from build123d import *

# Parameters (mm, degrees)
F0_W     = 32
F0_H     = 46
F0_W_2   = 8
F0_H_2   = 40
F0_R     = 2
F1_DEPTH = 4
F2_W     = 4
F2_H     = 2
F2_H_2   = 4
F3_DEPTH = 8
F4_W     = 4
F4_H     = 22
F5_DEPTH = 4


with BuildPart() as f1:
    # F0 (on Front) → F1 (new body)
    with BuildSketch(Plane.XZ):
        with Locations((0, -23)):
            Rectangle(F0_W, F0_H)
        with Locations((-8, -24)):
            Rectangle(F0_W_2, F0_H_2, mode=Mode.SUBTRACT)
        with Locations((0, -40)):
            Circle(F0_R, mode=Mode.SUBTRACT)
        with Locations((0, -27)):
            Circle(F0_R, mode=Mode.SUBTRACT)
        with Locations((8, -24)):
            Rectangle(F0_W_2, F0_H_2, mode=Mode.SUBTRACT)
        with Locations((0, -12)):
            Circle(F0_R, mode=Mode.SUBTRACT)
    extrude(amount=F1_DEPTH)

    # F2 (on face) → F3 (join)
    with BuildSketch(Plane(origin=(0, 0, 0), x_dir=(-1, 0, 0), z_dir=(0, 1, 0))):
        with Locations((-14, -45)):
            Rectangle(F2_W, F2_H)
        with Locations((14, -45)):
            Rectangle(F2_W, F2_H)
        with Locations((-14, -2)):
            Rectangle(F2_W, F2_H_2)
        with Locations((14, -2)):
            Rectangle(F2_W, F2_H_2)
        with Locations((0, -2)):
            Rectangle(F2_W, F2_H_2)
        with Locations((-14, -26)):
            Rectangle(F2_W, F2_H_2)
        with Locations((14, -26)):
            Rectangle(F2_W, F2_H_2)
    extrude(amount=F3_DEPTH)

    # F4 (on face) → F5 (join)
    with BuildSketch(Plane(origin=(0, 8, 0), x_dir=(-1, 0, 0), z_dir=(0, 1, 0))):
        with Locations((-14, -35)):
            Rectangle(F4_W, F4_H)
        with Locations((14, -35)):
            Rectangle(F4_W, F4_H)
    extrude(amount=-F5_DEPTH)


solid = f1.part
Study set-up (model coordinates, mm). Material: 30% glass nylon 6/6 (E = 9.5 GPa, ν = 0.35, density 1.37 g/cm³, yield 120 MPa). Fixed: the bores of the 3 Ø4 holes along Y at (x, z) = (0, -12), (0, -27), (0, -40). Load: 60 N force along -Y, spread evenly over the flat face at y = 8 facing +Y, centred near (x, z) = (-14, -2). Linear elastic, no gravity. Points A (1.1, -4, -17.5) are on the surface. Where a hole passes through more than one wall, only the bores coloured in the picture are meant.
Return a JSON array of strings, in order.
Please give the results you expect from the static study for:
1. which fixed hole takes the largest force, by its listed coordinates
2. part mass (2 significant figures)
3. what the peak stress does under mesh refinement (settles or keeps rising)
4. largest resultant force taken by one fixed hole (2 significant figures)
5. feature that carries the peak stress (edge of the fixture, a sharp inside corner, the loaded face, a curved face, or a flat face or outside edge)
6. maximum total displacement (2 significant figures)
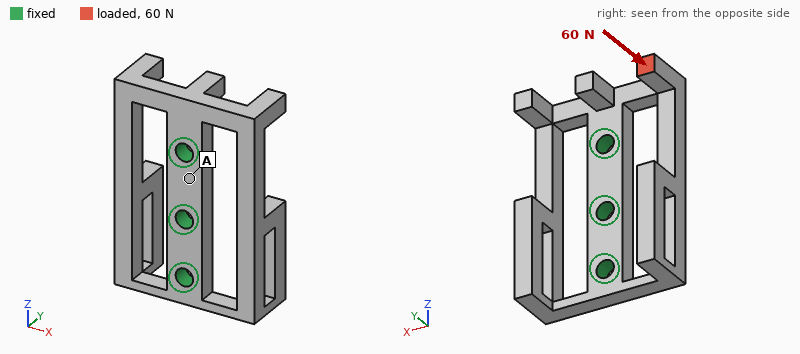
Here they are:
["(0, -12)", "6.1 g", "keeps rising", "61 N", "edge of the fixture", "0.53 mm"]
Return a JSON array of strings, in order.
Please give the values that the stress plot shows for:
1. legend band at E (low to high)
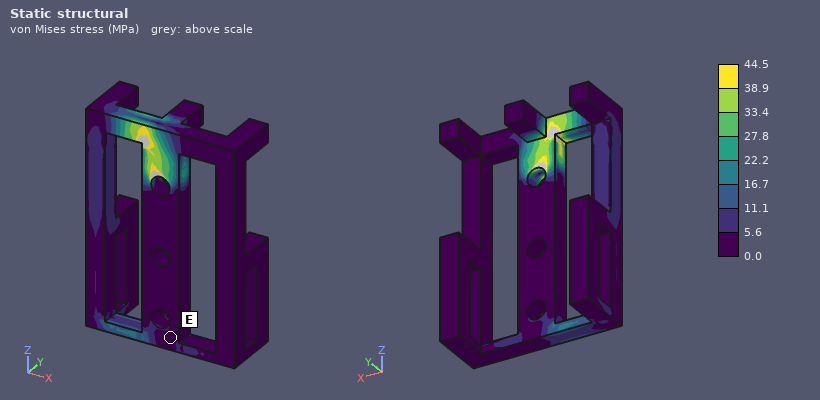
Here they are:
["0.0 to 5.6 MPa"]
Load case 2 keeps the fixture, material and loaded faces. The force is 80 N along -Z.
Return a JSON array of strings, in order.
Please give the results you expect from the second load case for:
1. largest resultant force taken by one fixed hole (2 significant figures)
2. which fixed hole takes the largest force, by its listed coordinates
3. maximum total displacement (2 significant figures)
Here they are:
["59 N", "(0, -12)", "0.60 mm"]
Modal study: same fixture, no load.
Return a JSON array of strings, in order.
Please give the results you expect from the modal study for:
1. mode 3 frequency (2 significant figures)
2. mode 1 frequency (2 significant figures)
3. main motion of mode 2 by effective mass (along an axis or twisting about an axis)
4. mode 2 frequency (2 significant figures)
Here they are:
["2500 Hz", "1500 Hz", "along Y", "1700 Hz"]
